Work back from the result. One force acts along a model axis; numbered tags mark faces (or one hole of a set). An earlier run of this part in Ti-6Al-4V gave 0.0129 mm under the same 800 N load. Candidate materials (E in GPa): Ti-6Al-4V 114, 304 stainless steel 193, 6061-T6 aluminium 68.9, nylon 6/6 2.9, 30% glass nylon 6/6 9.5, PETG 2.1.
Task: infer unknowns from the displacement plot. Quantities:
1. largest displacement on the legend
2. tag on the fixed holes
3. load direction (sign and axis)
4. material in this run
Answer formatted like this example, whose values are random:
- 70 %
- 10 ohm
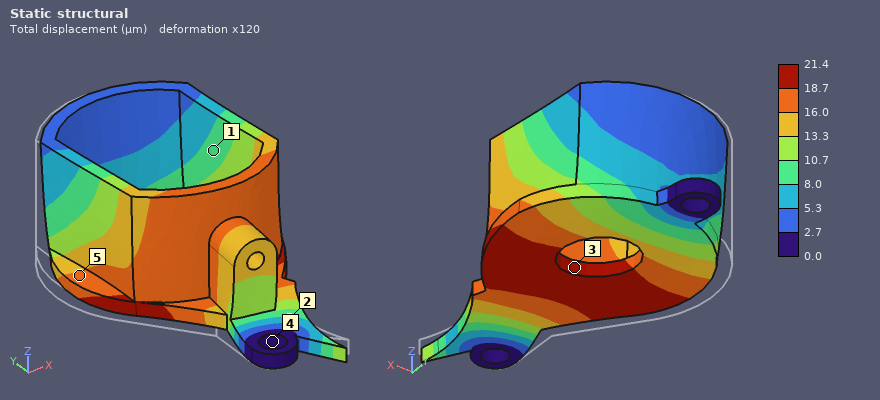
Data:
- 21.4 µm
- 4
- +X
- 6061-T6 aluminium
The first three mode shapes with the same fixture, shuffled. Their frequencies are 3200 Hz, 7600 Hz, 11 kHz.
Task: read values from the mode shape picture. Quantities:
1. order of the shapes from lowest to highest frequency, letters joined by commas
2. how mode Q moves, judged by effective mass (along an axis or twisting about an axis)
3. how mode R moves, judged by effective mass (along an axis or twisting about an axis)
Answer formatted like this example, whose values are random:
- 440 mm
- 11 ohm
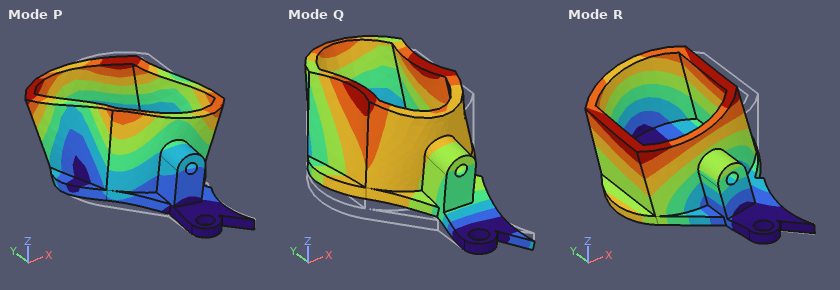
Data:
- R, Q, P
- along Z
- along X
